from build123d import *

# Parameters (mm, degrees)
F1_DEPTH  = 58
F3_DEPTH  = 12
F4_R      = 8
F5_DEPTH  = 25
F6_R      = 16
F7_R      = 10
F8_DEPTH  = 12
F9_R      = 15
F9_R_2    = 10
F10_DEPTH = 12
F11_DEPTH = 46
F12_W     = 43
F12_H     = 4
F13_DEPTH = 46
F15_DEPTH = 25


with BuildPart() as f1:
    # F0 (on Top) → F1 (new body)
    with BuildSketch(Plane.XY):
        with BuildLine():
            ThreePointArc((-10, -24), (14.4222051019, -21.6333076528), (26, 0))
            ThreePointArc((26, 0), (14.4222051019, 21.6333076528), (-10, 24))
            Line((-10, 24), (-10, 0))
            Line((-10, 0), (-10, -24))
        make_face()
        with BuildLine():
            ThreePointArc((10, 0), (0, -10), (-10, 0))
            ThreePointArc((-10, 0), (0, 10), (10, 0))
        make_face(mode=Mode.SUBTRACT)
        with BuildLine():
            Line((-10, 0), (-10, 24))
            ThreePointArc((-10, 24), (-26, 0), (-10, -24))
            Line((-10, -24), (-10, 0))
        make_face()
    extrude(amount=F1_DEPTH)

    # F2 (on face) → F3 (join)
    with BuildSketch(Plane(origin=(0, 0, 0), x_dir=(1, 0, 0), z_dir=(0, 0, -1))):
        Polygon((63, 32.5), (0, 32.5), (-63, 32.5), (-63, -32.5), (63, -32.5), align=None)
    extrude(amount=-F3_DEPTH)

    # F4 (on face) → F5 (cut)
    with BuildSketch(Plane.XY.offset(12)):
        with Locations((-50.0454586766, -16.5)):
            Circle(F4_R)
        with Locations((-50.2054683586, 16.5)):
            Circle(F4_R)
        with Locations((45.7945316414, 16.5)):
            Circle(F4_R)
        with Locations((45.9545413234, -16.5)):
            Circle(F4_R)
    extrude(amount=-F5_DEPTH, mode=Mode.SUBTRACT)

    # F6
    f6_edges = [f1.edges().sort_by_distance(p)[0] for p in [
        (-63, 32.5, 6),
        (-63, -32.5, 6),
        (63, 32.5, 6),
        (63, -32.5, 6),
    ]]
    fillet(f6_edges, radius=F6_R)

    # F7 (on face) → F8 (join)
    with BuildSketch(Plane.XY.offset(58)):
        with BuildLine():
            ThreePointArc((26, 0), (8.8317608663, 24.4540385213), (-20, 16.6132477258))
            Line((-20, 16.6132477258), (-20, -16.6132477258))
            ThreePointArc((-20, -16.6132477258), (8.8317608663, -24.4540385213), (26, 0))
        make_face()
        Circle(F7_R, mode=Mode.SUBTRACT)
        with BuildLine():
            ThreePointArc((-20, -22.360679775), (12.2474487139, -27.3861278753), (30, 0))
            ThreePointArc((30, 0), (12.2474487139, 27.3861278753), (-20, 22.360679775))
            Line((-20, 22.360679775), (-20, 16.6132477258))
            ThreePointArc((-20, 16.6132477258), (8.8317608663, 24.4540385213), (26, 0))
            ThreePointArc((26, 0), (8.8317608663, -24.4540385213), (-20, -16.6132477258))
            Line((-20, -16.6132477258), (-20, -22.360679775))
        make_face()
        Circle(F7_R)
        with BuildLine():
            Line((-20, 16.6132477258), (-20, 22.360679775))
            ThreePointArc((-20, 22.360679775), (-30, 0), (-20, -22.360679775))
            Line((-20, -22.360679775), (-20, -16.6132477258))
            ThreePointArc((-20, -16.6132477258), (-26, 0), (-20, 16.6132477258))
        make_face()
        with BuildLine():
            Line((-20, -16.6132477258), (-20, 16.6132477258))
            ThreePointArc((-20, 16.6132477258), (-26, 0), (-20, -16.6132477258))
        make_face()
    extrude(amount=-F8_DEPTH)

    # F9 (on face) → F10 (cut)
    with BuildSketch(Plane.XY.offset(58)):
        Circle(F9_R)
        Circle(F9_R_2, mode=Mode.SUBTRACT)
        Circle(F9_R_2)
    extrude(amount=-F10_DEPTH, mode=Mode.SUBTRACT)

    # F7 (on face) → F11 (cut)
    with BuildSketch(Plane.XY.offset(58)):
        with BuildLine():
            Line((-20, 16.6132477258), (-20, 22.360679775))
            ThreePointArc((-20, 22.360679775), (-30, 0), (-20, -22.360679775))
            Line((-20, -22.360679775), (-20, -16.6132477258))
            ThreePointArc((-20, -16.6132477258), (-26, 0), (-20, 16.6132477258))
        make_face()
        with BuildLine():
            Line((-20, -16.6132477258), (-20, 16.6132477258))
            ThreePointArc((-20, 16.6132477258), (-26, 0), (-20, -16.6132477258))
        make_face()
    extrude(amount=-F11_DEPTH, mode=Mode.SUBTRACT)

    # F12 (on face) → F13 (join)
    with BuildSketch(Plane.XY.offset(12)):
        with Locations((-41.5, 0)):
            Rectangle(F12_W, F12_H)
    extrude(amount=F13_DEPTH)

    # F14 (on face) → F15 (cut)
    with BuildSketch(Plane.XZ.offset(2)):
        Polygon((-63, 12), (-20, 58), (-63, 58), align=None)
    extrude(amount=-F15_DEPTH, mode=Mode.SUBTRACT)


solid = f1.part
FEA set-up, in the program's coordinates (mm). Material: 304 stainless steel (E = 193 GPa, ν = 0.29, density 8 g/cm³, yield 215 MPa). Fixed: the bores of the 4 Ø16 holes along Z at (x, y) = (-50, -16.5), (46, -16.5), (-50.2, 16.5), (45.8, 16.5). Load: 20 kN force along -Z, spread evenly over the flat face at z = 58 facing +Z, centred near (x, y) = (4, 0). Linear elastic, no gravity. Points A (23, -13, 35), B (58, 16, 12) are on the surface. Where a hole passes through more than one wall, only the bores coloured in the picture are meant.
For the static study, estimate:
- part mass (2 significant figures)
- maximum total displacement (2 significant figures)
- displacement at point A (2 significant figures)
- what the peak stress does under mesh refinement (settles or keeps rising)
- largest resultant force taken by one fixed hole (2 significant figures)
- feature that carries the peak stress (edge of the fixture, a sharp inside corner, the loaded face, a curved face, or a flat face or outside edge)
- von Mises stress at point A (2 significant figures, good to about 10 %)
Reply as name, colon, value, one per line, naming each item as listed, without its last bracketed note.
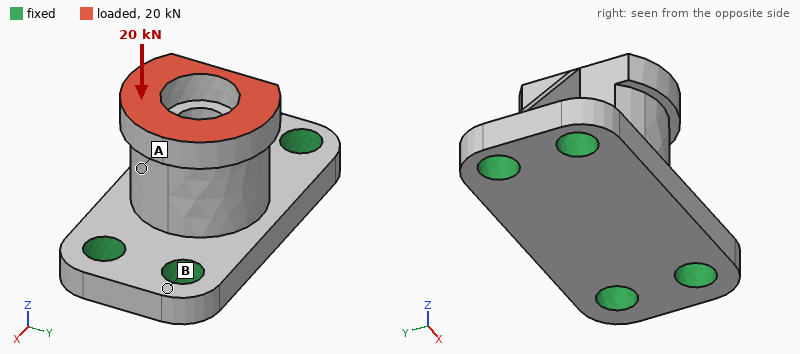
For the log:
part mass: 1.3 kg
maximum total displacement: 19 µm
displacement at point A: 16 µm
what the peak stress does under mesh refinement: keeps rising
largest resultant force taken by one fixed hole: 6.4 kN
feature that carries the peak stress: edge of the fixture
von Mises stress at point A: 20 MPa
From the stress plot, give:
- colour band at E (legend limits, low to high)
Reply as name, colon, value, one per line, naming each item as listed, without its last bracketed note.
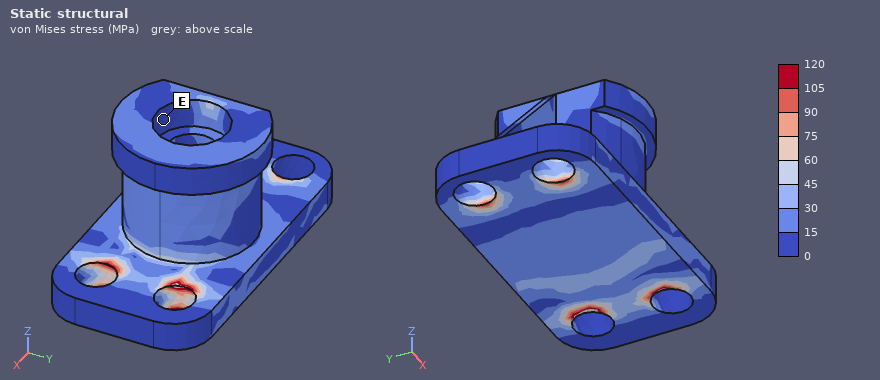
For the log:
colour band at E: 0 to 15 MPa
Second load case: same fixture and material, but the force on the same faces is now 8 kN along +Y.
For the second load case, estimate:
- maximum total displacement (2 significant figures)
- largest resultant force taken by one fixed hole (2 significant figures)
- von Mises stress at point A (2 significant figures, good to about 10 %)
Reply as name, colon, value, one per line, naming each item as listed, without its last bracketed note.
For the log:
maximum total displacement: 66 µm
largest resultant force taken by one fixed hole: 6.7 kN
von Mises stress at point A: 15 MPa
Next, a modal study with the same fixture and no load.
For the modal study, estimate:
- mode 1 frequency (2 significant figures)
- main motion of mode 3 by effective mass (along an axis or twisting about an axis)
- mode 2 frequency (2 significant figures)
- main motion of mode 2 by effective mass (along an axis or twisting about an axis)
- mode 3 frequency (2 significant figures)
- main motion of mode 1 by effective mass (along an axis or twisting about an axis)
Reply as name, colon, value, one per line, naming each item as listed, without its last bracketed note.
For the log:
mode 1 frequency: 3400 Hz
main motion of mode 3 by effective mass: along X
mode 2 frequency: 6100 Hz
main motion of mode 2 by effective mass: along Z
mode 3 frequency: 6800 Hz
main motion of mode 1 by effective mass: along Y
